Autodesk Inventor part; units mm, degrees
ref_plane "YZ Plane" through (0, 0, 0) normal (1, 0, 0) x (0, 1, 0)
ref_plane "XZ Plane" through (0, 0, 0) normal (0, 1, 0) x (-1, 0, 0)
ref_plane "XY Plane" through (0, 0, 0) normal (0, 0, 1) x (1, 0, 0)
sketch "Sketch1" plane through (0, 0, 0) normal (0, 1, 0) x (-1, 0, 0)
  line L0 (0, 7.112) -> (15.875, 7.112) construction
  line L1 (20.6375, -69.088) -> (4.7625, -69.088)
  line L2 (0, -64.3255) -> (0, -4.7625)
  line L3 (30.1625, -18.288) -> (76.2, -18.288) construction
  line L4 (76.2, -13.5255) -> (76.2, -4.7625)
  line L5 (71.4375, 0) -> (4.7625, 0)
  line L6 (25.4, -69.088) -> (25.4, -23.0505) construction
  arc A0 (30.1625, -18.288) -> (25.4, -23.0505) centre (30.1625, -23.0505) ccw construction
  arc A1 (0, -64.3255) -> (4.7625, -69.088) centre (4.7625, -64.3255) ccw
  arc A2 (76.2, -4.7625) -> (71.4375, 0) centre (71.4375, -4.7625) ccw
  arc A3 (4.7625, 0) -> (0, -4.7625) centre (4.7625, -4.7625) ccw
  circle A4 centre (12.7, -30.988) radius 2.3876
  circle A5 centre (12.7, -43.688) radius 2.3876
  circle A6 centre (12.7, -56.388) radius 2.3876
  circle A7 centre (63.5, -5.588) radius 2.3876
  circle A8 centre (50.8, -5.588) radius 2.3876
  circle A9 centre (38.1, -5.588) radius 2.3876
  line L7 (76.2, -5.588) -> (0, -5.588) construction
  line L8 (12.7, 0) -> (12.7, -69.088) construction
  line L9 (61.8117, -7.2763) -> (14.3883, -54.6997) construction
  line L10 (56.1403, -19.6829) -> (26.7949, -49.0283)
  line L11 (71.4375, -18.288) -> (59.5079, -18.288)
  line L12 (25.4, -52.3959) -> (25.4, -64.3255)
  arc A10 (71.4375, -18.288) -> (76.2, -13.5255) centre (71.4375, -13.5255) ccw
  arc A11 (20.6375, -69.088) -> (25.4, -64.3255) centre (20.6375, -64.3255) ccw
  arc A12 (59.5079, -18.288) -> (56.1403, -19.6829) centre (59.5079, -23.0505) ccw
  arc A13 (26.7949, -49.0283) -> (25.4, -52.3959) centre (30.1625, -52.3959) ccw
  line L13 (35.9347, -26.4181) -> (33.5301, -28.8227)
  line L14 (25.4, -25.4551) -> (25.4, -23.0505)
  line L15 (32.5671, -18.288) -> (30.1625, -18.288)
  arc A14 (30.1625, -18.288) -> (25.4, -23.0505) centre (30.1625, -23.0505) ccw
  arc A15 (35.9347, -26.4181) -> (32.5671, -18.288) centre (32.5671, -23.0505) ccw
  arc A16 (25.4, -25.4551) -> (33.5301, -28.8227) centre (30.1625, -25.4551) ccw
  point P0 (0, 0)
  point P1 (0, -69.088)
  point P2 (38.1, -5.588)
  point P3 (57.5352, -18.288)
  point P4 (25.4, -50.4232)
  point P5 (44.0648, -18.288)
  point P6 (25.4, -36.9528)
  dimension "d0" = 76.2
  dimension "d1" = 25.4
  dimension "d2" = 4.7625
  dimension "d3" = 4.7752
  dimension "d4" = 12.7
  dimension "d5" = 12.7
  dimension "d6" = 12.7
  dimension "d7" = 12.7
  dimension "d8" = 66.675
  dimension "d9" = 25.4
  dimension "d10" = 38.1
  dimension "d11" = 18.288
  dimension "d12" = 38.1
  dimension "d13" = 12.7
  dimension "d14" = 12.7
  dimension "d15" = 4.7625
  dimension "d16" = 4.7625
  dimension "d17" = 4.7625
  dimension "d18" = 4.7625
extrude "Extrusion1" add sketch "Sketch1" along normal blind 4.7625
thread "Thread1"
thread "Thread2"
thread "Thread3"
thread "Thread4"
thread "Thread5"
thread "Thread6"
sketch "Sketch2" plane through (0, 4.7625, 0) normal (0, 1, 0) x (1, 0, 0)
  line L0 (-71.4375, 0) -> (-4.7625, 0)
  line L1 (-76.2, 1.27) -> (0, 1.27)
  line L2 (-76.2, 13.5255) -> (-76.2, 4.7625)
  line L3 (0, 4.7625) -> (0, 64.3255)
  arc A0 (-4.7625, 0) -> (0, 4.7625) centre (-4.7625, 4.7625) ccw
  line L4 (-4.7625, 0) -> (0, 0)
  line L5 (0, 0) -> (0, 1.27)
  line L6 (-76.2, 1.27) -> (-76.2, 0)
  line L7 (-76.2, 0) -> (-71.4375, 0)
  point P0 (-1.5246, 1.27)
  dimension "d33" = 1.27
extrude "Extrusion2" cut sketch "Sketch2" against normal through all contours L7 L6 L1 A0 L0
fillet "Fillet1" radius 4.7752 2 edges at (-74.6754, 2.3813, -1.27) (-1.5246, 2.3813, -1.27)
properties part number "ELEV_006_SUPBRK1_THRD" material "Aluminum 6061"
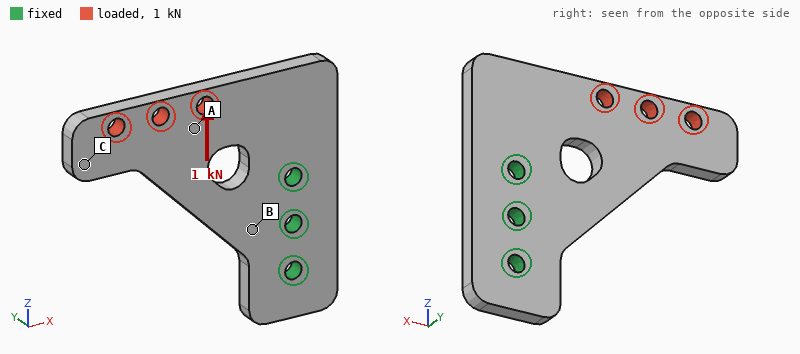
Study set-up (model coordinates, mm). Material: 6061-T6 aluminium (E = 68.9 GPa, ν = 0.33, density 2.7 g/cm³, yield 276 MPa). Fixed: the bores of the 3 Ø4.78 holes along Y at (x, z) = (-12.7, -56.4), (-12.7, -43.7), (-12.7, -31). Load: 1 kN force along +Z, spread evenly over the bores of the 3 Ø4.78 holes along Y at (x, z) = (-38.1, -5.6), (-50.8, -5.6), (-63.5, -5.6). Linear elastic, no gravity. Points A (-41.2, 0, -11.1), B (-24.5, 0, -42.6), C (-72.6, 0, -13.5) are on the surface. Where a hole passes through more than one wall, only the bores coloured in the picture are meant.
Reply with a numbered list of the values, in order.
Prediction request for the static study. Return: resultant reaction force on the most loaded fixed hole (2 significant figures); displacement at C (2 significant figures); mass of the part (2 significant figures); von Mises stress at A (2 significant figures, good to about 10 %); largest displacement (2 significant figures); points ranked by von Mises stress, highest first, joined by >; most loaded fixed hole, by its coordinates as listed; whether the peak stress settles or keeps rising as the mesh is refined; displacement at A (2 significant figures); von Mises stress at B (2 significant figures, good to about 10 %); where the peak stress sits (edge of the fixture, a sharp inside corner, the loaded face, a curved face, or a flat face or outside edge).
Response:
1. 1.6 kN
2. 72 µm
3. 37 g
4. 14 MPa
5. 80 µm
6. B > A > C
7. (-12.7, -31)
8. keeps rising
9. 35 µm
10. 22 MPa
11. edge of the fixture
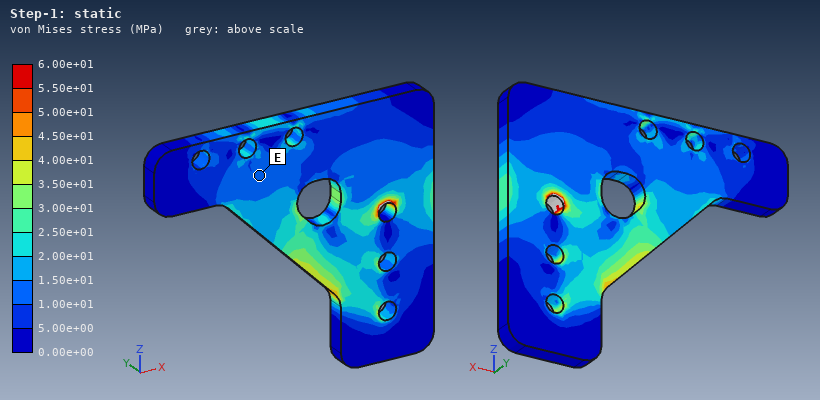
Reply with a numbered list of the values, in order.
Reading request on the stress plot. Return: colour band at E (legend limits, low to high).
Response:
1. 1.00e+01 to 1.50e+01 MPa
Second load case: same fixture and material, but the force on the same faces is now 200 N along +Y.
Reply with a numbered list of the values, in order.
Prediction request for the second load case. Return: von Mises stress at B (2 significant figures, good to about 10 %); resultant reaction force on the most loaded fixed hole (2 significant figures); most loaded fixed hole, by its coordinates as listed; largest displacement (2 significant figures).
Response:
1. 36 MPa
2. 340 N
3. (-12.7, -31)
4. 0.58 mm
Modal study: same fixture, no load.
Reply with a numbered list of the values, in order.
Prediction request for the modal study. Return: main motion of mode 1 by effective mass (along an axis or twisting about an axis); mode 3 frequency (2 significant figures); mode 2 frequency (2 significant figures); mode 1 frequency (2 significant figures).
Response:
1. along Y
2. 5500 Hz
3. 3700 Hz
4. 1100 Hz
